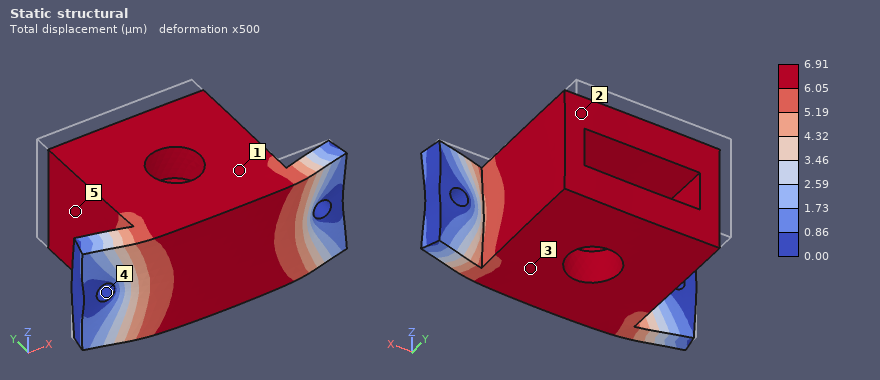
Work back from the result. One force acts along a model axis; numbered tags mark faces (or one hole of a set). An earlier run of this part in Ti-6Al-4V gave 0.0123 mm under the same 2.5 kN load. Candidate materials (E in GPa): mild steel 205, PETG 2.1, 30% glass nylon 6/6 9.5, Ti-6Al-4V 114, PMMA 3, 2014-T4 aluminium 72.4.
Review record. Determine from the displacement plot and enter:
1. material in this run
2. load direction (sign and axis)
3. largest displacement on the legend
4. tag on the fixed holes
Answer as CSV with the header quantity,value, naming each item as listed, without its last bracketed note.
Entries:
quantity,value
material in this run,mild steel
load direction,-Y
largest displacement on the legend,6.91 µm
tag on the fixed holes,4
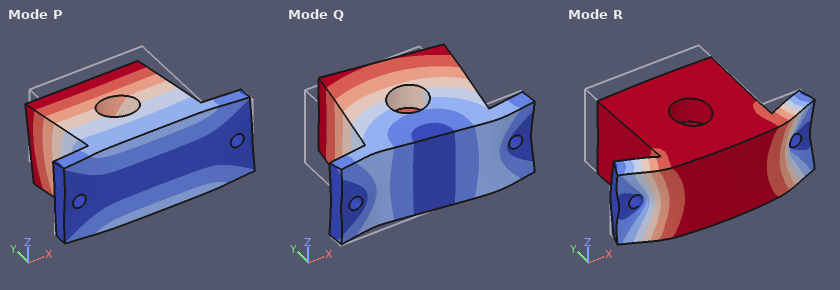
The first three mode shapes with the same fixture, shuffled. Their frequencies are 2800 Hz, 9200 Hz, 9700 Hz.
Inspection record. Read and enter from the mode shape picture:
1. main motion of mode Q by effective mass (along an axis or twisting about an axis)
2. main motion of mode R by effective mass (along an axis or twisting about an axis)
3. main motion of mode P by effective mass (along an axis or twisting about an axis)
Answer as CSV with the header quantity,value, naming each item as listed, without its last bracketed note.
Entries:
quantity,value
main motion of mode Q by effective mass,along X
main motion of mode R by effective mass,along Y
main motion of mode P by effective mass,along Z
